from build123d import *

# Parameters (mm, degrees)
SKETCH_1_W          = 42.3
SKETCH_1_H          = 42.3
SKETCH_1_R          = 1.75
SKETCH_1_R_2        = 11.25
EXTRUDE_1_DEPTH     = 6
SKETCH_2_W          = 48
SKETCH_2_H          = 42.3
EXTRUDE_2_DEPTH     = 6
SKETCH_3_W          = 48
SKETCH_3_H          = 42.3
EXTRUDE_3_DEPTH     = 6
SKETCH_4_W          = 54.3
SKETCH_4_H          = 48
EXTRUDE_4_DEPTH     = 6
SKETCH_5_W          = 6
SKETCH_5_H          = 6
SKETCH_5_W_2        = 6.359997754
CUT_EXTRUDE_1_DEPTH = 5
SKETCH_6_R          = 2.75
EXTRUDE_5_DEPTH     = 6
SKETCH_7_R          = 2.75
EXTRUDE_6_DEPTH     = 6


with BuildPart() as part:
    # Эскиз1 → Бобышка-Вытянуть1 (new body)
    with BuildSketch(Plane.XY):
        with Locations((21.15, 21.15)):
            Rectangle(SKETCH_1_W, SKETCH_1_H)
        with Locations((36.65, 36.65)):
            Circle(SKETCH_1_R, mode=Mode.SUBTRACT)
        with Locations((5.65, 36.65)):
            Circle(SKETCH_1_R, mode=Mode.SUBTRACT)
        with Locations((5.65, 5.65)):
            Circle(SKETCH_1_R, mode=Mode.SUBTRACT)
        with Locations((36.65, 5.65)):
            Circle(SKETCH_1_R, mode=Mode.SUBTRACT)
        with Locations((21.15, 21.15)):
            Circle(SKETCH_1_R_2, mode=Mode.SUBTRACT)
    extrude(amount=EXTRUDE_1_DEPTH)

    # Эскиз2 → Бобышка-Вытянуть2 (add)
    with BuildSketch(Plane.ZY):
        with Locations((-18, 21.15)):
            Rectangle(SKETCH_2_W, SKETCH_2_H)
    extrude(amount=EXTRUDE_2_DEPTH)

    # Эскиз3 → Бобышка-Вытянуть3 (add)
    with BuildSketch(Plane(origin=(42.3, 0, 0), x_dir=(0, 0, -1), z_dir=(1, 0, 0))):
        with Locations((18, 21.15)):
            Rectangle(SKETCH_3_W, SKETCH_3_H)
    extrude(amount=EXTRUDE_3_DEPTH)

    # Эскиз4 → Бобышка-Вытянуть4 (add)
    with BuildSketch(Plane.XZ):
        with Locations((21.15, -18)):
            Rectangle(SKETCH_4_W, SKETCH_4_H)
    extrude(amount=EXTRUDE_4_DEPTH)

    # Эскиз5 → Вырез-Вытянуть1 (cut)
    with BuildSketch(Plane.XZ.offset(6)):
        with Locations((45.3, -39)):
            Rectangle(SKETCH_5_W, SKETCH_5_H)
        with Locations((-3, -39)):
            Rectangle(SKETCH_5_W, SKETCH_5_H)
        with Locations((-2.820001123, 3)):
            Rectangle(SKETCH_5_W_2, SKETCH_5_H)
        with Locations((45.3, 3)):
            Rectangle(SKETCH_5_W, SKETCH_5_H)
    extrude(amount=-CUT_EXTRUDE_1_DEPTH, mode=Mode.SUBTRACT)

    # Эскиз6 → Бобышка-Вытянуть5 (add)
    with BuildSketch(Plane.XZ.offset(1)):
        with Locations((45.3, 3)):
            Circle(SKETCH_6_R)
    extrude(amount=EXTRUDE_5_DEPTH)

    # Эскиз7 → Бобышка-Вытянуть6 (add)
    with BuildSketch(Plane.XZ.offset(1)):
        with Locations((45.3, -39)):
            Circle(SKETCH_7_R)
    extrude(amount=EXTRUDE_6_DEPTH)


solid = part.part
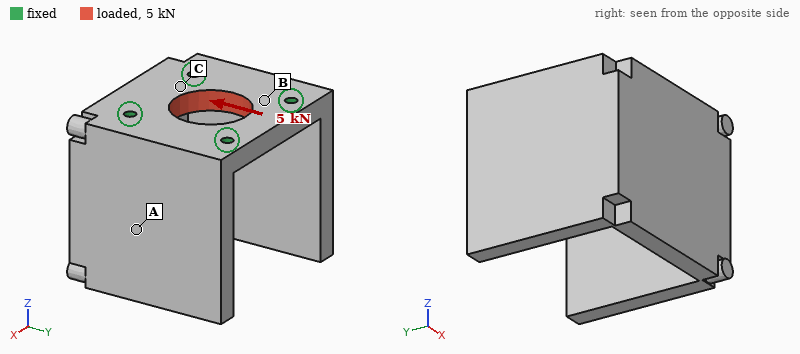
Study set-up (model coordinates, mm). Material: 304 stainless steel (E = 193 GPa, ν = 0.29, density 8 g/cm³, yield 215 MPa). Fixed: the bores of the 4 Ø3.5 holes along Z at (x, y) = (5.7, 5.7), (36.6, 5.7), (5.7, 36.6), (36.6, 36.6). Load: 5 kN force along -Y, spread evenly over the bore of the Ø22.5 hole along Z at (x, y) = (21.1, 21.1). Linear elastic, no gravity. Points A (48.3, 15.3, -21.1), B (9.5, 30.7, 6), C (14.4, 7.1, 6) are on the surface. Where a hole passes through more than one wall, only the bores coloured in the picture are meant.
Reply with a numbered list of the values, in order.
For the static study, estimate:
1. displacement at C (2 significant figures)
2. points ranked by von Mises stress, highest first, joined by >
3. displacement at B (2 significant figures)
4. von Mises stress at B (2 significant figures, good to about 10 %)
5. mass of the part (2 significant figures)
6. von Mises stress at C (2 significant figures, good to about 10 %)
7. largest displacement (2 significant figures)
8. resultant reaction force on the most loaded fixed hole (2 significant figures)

1. 1.1 µm
2. B > C > A
3. 0.89 µm
4. 18 MPa
5. 380 g
6. 11 MPa
7. 2.6 µm
8. 1.3 kN
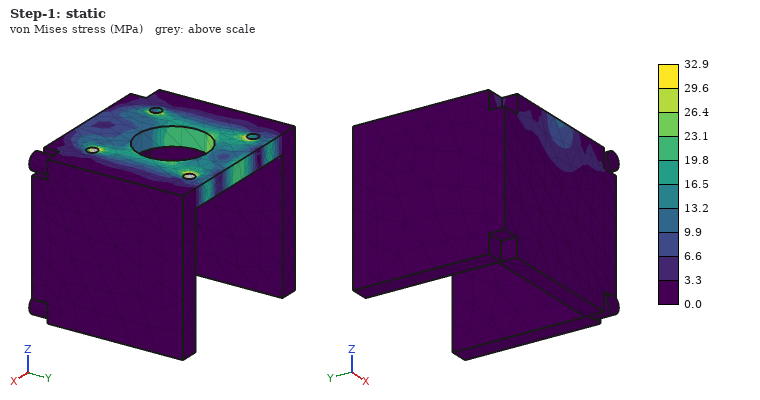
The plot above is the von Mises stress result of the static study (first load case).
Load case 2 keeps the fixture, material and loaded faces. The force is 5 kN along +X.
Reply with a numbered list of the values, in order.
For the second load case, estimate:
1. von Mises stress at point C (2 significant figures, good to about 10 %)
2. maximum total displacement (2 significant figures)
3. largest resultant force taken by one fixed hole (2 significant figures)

1. 14 MPa
2. 1.7 µm
3. 1.3 kN
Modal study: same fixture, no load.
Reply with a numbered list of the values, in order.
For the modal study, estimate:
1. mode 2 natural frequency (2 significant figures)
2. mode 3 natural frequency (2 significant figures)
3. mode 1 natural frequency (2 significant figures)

1. 3300 Hz
2. 5400 Hz
3. 3300 Hz
